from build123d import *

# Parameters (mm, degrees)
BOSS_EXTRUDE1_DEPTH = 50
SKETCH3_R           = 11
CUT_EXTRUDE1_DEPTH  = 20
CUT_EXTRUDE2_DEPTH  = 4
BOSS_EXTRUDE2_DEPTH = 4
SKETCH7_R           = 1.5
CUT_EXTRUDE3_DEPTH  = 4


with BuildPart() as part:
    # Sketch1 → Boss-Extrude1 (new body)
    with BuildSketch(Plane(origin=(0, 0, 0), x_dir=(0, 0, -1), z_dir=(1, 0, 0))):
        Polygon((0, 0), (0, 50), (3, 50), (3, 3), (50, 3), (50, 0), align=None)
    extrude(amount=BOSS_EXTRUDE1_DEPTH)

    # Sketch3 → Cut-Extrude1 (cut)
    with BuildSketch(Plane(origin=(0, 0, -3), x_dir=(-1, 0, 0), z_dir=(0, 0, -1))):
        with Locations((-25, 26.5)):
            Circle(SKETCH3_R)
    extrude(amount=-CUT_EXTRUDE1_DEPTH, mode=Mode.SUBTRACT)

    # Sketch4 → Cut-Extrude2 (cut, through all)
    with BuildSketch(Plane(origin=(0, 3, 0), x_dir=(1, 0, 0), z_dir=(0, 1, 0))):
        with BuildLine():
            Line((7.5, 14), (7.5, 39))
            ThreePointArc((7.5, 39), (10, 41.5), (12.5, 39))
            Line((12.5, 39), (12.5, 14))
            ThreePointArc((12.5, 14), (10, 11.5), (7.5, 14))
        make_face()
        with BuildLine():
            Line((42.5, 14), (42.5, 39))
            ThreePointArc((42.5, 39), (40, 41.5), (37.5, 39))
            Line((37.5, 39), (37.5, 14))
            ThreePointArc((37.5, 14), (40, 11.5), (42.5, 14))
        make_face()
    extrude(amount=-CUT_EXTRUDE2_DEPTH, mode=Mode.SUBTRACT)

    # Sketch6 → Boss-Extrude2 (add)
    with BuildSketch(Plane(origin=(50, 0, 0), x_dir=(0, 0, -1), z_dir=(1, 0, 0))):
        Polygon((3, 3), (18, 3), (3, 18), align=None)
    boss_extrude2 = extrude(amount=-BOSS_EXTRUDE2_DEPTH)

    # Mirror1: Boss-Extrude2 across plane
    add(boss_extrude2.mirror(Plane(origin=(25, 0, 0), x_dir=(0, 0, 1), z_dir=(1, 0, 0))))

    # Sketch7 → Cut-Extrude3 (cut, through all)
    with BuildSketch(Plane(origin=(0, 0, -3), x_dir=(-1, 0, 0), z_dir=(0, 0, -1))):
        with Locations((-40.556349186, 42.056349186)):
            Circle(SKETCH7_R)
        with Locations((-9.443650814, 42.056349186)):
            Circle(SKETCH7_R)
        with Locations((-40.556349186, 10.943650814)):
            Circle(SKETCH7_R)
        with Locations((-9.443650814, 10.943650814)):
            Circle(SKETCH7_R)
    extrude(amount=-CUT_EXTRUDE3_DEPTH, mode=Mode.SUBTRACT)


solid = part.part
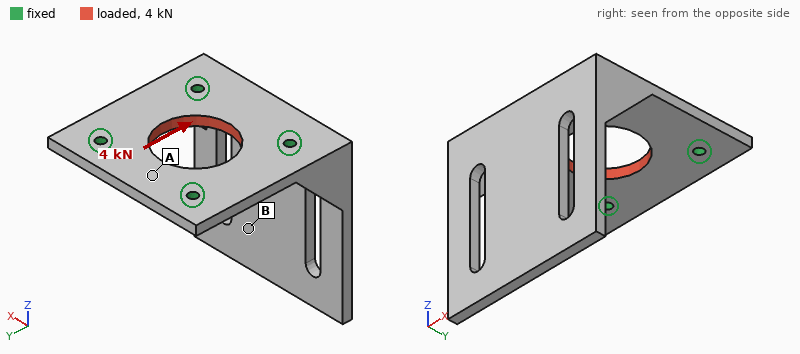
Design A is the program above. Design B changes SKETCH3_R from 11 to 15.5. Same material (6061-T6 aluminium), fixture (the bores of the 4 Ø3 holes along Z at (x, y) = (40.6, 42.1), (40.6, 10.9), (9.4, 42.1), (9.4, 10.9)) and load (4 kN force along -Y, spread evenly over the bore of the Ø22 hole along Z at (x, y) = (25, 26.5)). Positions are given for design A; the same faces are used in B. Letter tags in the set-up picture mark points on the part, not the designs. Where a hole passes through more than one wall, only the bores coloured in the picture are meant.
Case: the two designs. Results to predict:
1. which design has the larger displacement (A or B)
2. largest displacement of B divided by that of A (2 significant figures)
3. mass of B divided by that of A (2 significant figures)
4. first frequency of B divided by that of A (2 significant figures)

B
1.2
0.92
0.98
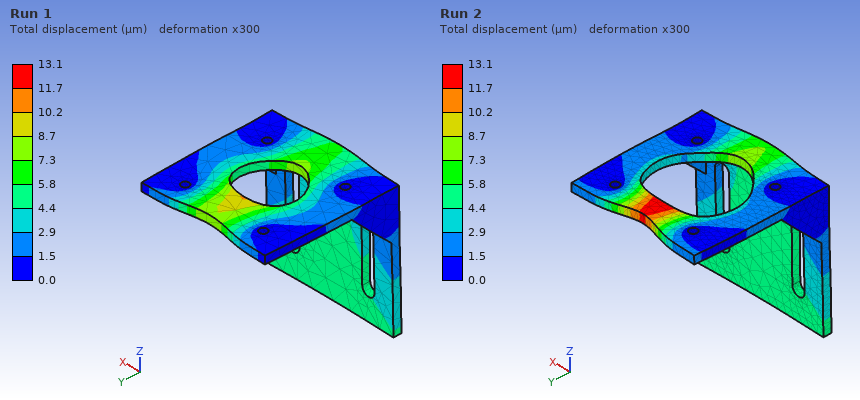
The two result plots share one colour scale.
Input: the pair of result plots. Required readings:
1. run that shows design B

Run 2
